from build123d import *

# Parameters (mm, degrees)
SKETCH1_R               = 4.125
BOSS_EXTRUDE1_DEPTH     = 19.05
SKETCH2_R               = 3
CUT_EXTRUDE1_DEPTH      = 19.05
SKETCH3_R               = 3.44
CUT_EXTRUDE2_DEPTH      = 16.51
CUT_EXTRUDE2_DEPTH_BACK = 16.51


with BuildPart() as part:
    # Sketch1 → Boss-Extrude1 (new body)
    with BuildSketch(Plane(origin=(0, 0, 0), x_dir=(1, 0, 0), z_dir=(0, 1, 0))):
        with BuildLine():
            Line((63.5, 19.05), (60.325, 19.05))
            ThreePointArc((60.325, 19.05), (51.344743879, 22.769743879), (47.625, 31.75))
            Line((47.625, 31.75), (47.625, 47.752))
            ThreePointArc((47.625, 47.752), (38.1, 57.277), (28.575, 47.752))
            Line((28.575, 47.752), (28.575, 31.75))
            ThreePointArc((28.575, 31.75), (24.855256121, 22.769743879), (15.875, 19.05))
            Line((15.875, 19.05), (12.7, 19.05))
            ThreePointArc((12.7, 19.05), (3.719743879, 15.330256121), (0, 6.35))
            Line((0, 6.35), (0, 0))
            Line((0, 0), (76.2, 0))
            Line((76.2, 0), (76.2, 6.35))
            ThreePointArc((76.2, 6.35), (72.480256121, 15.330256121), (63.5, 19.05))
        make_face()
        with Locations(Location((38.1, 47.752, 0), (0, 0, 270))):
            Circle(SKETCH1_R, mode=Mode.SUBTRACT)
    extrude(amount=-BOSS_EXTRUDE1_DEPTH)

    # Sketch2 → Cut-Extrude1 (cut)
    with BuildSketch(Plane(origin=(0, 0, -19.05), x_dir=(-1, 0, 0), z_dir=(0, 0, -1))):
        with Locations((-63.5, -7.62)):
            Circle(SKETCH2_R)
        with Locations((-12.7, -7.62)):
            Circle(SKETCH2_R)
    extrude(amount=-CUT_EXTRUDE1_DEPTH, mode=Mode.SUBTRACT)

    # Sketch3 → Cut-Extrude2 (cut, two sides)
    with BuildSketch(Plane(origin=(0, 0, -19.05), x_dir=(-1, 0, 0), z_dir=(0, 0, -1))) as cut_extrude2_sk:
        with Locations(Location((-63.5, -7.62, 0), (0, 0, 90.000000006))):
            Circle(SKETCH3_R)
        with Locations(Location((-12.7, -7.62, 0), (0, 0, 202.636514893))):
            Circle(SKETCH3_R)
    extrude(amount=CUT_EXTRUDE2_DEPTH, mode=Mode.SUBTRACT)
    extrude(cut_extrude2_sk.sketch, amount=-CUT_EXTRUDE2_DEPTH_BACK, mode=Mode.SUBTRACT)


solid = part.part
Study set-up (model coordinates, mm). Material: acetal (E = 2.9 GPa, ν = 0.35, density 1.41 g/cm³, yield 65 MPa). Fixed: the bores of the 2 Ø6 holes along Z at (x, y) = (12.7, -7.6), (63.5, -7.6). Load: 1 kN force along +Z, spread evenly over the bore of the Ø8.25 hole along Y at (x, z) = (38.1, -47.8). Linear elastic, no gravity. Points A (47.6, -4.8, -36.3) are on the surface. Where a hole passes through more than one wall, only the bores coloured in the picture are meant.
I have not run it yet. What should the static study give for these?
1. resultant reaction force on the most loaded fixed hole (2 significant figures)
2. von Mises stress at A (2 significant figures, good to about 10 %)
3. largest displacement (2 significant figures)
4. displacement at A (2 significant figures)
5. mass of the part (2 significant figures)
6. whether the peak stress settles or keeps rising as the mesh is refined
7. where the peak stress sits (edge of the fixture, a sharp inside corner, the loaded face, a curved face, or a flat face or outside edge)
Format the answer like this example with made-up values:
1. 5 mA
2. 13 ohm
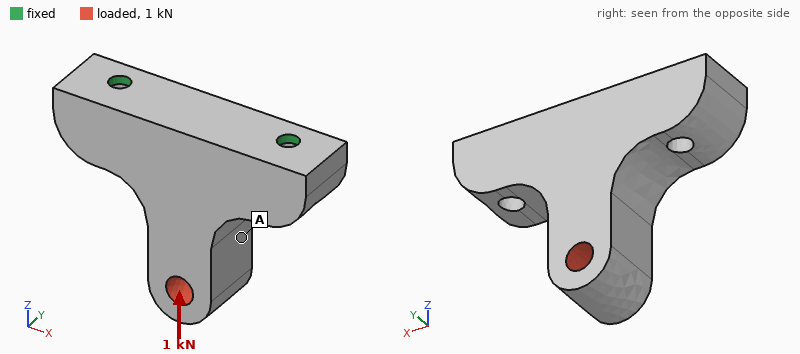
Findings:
1. 580 N
2. 3.1 MPa
3. 0.29 mm
4. 0.17 mm
5. 54 g
6. keeps rising
7. edge of the fixture
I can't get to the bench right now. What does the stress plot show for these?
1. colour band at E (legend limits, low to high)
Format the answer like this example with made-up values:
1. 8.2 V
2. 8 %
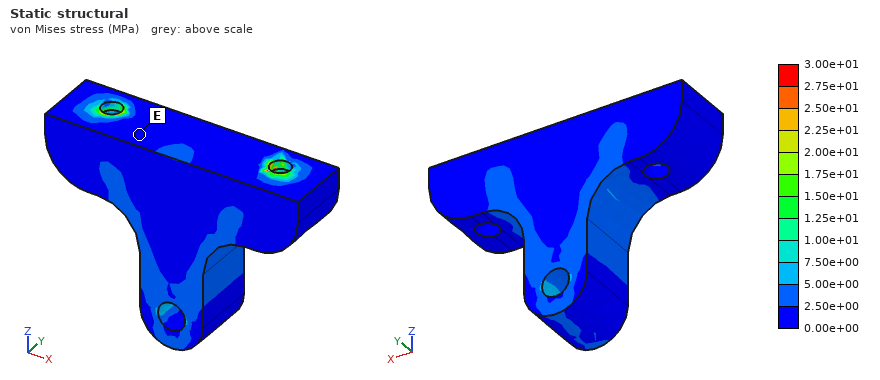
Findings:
1. 0.00e+00 to 2.50e+00 MPa
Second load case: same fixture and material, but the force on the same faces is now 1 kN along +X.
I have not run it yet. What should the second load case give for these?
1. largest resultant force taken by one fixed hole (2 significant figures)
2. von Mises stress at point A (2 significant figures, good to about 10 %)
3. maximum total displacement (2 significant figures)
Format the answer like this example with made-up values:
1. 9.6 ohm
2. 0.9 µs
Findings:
1. 1.0 kN
2. 11 MPa
3. 0.57 mm
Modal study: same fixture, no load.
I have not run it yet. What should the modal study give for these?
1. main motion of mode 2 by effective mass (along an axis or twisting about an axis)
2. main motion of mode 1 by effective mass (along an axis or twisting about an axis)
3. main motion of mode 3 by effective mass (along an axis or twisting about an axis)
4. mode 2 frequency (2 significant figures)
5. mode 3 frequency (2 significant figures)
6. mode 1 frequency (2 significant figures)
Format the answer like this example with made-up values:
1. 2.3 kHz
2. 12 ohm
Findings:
1. along X
2. along Y
3. along Z
4. 2500 Hz
5. 3400 Hz
6. 570 Hz
